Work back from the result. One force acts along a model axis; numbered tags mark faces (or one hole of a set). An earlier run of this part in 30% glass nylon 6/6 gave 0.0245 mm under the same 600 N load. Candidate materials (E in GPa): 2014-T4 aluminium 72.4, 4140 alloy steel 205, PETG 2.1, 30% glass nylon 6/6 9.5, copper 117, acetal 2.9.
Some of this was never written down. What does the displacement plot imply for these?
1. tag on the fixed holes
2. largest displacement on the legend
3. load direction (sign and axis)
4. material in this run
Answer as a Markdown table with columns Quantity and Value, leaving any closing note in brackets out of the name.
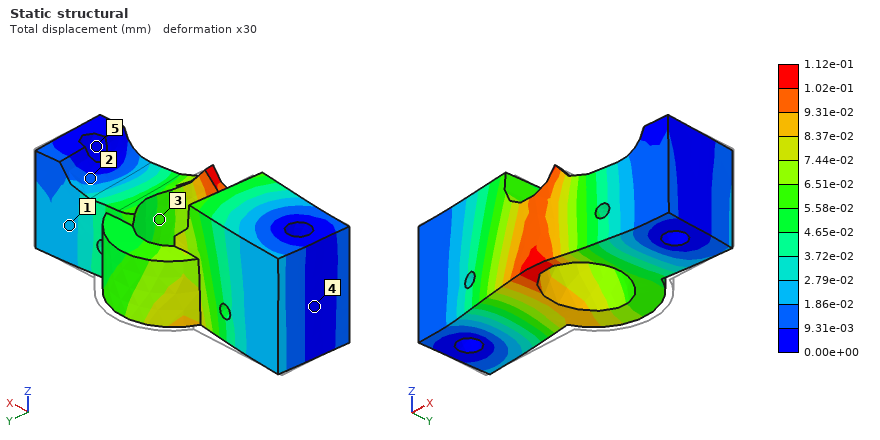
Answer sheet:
| Quantity | Value |
|---|---|
| tag on the fixed holes | 5 |
| largest displacement on the legend | 1.12e-01 mm |
| load direction | -Y |
| material in this run | PETG |
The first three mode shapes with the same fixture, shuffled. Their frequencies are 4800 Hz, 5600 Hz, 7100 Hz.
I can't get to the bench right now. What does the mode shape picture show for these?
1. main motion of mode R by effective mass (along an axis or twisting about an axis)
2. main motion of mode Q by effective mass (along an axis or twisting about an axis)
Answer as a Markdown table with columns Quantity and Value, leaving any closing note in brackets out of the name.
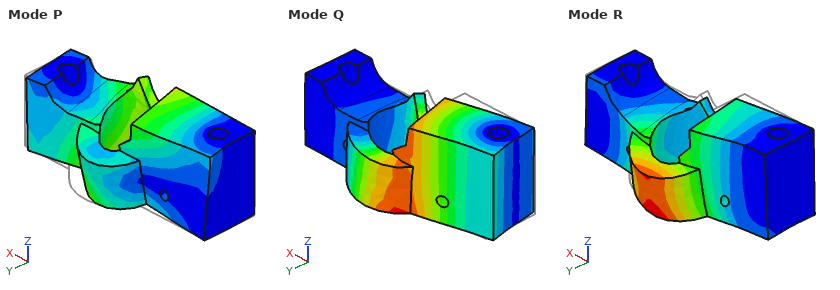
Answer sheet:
| Quantity | Value |
|---|---|
| main motion of mode R by effective mass | along Z |
| main motion of mode Q by effective mass | along Y |
